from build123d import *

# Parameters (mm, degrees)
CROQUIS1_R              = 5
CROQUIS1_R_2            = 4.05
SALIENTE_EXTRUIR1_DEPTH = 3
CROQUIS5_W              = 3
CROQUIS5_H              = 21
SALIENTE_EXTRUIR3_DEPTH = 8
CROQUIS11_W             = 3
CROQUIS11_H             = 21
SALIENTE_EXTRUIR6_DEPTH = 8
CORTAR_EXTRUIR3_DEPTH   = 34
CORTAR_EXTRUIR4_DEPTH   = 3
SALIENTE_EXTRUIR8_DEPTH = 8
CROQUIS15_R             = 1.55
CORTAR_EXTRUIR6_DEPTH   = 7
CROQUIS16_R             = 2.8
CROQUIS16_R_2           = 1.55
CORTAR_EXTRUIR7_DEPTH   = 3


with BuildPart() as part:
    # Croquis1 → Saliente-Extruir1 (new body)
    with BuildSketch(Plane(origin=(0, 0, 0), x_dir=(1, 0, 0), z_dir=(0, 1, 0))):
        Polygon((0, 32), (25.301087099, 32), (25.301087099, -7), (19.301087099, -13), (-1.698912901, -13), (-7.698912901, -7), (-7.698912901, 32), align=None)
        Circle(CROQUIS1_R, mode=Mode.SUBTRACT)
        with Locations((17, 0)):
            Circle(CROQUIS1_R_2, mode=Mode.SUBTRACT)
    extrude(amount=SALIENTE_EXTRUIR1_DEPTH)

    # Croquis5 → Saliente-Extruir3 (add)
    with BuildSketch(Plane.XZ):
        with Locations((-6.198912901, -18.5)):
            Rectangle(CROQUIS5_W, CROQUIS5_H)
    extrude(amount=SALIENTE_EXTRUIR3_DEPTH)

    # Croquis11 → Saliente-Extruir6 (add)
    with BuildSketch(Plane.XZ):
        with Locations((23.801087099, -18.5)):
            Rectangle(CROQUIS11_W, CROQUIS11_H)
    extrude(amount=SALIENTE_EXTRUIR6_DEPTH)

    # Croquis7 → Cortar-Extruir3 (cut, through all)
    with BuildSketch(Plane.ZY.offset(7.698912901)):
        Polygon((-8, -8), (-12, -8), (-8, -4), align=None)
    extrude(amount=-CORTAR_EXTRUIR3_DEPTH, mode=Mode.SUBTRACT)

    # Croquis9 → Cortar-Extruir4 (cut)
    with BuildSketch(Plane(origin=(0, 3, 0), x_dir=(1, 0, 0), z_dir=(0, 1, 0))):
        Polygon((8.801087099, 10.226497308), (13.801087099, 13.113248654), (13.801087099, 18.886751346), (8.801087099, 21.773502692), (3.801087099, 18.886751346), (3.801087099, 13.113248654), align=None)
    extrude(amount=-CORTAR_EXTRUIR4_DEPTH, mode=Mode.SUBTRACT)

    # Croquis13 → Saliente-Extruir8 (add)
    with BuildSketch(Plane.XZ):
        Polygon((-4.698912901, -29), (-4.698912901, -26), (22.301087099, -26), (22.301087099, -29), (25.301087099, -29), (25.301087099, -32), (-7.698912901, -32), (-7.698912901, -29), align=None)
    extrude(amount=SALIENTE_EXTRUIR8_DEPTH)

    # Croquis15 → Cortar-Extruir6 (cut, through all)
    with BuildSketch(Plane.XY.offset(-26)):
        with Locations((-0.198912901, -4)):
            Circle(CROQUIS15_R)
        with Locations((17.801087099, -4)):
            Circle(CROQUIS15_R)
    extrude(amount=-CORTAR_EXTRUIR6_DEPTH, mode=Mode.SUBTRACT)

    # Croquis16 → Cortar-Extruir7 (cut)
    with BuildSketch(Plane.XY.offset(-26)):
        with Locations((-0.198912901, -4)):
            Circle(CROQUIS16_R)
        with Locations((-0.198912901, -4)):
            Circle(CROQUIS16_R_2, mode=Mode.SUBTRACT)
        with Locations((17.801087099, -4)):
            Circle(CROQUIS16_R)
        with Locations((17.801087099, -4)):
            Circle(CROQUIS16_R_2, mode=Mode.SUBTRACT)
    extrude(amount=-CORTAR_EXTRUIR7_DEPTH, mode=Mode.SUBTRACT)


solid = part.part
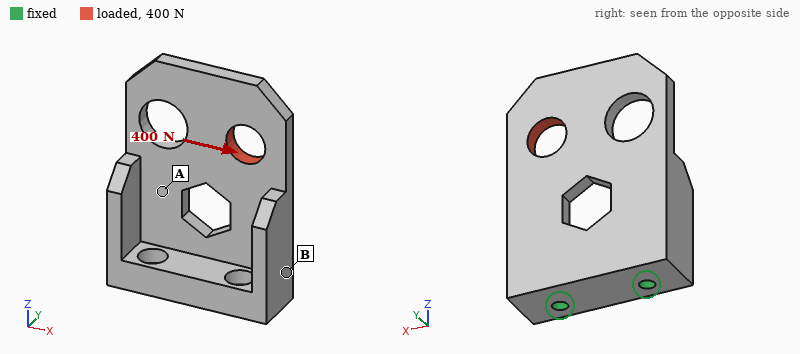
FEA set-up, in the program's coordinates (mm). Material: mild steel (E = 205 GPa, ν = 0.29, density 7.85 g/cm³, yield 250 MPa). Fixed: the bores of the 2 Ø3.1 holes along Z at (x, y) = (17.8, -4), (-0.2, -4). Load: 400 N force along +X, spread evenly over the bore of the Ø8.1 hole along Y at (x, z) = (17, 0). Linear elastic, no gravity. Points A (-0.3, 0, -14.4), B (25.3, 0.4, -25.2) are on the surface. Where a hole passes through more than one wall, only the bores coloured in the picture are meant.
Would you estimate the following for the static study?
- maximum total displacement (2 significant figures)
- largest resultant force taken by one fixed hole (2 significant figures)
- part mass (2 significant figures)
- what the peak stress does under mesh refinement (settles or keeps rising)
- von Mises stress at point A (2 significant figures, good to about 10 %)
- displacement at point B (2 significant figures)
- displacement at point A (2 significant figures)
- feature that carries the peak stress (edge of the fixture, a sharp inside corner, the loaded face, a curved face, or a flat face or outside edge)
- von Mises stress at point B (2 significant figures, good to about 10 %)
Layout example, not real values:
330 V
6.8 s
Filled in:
19 µm
640 N
46 g
keeps rising
25 MPa
4.5 µm
7.0 µm
edge of the fixture
13 MPa
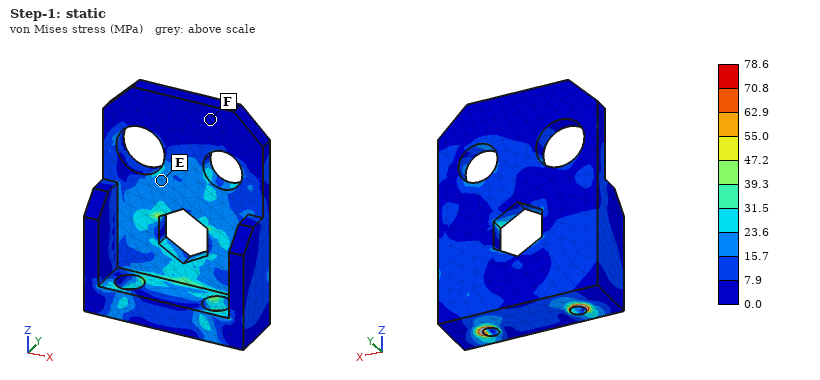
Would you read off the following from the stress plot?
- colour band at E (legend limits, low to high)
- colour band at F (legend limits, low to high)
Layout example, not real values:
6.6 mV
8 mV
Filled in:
15.7 to 23.6 MPa
0.0 to 7.9 MPa
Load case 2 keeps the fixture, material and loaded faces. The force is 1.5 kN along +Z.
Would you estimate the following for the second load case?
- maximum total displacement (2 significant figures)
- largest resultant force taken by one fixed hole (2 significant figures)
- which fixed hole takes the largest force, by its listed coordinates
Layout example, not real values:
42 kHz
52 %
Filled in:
55 µm
1.4 kN
(17.8, -4)
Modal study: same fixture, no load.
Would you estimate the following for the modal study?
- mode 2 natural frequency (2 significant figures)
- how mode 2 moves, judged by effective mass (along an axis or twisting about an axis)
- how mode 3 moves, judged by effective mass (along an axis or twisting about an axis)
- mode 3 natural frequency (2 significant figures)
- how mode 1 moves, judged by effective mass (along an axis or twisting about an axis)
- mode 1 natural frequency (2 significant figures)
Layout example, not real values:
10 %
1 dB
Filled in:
5000 Hz
along X
along Y
7500 Hz
along Y
2300 Hz
